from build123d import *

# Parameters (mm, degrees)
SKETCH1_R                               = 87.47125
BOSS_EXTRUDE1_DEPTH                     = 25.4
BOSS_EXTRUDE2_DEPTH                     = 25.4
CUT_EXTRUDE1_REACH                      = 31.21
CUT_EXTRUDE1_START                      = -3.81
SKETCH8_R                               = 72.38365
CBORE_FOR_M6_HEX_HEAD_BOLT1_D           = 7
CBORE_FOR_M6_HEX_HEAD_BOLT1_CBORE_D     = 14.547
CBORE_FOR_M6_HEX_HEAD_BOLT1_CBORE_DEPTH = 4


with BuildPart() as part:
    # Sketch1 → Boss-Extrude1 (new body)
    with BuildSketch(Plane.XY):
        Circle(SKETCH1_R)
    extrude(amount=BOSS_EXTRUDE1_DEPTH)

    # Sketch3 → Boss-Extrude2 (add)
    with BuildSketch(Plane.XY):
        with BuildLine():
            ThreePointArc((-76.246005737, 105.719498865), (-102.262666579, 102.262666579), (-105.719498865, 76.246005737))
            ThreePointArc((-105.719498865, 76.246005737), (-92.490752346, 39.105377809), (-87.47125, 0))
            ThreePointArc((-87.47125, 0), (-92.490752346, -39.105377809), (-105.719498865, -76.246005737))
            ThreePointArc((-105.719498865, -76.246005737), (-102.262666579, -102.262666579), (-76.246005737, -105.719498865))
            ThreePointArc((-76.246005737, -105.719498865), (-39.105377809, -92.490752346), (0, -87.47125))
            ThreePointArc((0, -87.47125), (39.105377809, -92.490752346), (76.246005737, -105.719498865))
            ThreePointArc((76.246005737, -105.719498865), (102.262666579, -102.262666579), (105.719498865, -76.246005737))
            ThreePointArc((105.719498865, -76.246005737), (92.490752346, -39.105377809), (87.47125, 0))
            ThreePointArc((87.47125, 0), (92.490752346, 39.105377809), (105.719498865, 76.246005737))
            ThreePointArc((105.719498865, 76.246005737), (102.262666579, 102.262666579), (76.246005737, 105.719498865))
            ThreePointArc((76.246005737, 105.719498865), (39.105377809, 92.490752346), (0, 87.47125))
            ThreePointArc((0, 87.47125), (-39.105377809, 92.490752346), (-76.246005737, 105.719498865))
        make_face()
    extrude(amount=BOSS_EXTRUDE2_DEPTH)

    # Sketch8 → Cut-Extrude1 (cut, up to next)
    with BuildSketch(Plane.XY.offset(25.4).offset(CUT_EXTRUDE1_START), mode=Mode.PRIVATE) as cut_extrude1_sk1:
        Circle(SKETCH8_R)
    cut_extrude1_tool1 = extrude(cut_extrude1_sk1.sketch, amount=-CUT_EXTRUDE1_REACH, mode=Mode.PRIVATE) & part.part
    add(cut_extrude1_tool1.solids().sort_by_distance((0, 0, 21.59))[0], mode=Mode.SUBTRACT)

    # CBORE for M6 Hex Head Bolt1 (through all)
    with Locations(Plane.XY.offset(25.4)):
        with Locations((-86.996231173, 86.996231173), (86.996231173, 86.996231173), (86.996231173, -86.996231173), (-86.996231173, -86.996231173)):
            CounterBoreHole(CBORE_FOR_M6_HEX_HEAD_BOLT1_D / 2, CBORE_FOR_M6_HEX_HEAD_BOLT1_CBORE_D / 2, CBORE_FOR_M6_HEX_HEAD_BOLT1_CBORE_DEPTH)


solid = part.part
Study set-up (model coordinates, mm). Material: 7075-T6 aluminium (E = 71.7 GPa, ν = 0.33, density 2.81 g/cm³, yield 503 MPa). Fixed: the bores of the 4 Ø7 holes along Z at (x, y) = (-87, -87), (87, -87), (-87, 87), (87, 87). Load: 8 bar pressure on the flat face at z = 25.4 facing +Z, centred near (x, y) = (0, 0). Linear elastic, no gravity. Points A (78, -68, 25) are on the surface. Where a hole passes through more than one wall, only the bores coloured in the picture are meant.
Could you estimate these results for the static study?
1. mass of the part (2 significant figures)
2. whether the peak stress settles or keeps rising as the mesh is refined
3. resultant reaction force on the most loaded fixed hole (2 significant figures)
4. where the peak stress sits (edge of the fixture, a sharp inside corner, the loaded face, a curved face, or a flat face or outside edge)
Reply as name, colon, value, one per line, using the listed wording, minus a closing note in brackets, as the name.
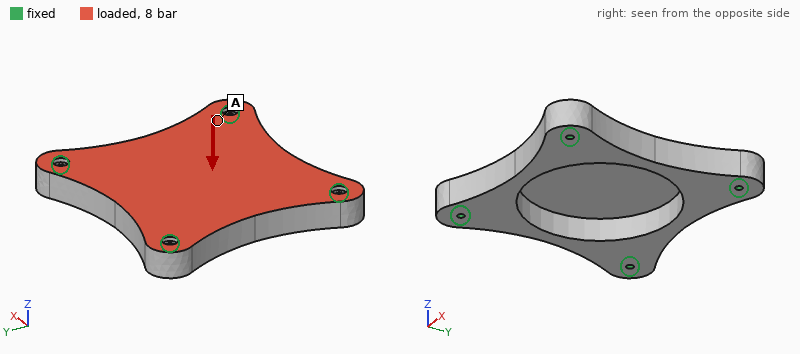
mass of the part: 1.7 kg
whether the peak stress settles or keeps rising as the mesh is refined: keeps rising
resultant reaction force on the most loaded fixed hole: 9.6 kN
where the peak stress sits: edge of the fixture
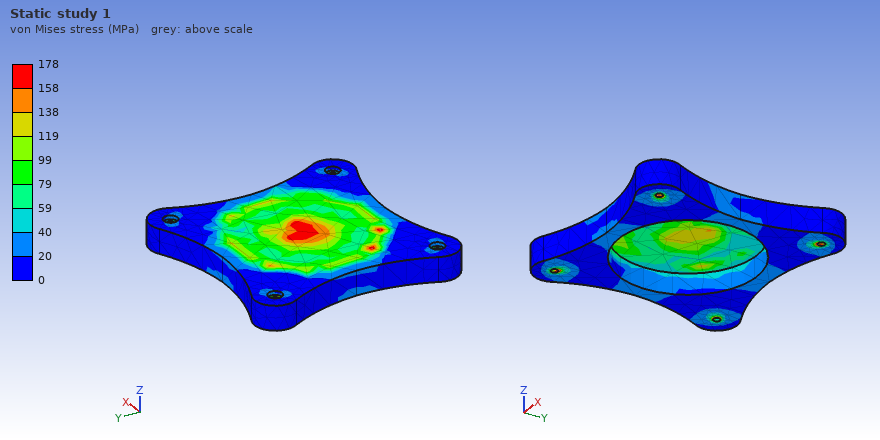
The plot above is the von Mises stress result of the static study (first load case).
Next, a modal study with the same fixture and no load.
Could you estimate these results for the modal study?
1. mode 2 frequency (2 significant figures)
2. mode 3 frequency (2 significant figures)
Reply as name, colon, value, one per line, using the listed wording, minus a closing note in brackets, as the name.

mode 2 frequency: 3300 Hz
mode 3 frequency: 3300 Hz
